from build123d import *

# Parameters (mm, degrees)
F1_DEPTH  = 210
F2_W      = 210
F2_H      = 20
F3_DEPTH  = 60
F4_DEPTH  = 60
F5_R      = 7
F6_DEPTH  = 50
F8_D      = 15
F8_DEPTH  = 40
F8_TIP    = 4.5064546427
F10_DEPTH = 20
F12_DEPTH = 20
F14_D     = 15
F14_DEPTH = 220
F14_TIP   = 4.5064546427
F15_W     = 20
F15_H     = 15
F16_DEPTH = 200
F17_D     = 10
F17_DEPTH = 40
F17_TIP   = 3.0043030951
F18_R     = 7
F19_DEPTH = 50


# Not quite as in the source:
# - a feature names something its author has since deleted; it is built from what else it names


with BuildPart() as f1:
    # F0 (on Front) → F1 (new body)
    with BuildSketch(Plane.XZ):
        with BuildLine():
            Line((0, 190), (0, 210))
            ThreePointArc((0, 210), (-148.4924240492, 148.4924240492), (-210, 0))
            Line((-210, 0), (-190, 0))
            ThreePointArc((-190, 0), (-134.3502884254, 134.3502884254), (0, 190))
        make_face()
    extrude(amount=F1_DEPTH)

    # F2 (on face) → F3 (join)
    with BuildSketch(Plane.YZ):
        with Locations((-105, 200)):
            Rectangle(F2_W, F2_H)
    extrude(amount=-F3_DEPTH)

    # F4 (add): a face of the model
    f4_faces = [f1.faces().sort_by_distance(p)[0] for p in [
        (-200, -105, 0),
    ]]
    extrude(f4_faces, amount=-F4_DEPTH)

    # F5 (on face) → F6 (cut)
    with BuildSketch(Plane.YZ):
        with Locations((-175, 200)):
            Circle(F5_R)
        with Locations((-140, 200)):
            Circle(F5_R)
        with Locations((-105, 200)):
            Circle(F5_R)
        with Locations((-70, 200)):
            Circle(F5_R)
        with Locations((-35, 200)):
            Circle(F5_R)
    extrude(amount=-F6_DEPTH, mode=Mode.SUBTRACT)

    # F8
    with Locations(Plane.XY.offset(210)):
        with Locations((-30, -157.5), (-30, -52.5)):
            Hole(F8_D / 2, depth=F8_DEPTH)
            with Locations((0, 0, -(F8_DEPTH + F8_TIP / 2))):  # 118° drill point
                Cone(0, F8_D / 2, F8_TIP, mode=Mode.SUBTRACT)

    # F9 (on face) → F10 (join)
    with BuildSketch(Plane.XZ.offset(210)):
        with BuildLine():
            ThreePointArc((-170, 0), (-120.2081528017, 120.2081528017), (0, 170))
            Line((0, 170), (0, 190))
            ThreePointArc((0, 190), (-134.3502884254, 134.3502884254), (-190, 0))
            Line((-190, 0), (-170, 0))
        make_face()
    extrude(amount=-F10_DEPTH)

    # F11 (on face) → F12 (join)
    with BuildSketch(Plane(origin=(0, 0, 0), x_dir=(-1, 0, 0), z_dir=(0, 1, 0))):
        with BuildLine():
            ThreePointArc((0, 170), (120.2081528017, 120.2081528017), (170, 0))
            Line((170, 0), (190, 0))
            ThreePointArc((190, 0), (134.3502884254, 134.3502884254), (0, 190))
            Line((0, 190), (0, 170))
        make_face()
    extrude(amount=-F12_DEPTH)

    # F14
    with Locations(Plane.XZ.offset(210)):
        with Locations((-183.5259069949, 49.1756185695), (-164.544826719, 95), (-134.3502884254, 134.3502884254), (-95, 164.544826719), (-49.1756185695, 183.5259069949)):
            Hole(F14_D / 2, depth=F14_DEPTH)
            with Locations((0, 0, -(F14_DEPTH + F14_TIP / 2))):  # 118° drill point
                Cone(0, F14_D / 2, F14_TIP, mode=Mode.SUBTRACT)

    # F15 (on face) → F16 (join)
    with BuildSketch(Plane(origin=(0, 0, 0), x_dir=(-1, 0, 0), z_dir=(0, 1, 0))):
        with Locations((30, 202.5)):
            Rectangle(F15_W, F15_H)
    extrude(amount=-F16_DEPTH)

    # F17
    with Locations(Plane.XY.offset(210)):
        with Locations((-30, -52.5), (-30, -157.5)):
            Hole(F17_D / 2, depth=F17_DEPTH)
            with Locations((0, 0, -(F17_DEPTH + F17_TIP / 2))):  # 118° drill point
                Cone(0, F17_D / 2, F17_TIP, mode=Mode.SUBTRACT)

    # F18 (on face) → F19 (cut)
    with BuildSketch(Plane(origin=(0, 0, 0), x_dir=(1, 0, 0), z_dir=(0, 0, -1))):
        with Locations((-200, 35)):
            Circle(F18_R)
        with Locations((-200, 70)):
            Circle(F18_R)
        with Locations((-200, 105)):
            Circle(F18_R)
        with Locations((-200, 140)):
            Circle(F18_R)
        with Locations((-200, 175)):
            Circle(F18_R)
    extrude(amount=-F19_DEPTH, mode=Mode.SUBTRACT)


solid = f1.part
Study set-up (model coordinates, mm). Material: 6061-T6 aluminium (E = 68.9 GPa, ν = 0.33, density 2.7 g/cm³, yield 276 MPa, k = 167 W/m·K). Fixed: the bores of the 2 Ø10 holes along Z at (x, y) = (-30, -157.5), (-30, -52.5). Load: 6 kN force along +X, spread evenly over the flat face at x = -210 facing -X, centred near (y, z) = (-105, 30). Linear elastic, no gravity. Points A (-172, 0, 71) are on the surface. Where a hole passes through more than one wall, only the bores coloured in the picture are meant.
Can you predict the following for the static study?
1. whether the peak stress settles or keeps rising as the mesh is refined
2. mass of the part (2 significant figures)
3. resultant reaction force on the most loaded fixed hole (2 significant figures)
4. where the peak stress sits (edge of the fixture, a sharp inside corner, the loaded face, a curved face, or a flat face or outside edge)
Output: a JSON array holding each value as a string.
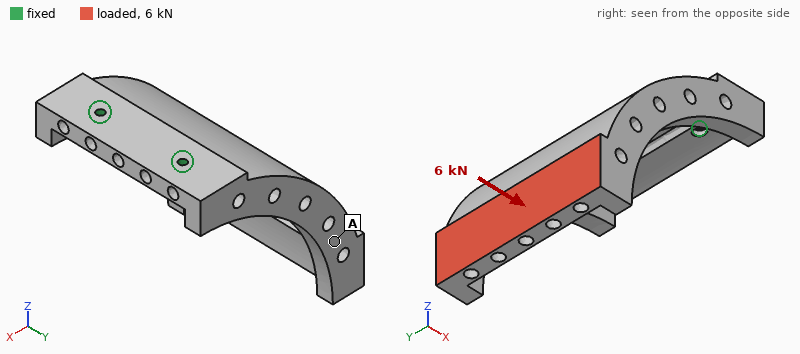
["keeps rising", "3.9 kg", "4.9 kN", "edge of the fixture"]
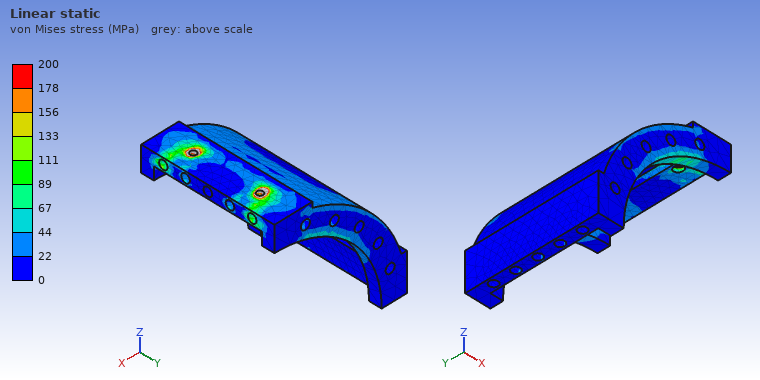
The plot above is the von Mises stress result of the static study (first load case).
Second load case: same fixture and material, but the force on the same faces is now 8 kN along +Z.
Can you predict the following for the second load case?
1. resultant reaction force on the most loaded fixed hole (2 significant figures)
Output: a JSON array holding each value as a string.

["5.7 kN"]
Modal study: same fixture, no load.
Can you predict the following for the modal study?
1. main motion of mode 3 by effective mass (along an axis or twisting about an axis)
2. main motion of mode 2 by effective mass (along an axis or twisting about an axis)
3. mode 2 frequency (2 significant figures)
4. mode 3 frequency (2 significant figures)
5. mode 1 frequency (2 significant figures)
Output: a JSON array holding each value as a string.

["along Y", "along Y", "420 Hz", "1000 Hz", "200 Hz"]
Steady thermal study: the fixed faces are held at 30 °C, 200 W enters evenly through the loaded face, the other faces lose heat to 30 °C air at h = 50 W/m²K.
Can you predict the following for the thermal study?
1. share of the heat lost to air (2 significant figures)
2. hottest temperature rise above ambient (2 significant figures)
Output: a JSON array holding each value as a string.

["75 %", "37 K"]
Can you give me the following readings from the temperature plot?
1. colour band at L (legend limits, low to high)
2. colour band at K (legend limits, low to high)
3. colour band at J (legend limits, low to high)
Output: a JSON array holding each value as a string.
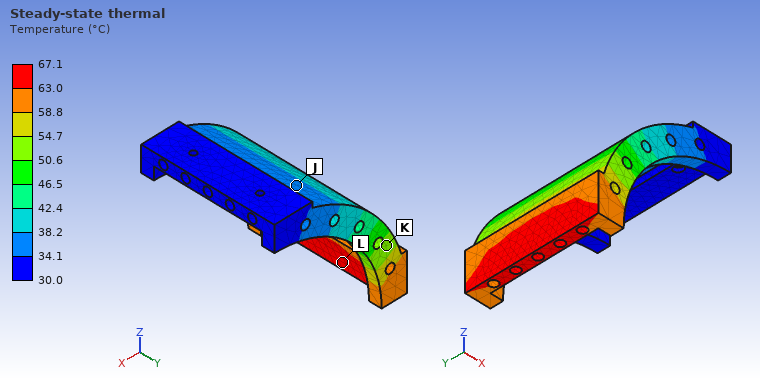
["63.0 to 67.1 °C", "50.6 to 54.7 °C", "34.1 to 38.2 °C"]
